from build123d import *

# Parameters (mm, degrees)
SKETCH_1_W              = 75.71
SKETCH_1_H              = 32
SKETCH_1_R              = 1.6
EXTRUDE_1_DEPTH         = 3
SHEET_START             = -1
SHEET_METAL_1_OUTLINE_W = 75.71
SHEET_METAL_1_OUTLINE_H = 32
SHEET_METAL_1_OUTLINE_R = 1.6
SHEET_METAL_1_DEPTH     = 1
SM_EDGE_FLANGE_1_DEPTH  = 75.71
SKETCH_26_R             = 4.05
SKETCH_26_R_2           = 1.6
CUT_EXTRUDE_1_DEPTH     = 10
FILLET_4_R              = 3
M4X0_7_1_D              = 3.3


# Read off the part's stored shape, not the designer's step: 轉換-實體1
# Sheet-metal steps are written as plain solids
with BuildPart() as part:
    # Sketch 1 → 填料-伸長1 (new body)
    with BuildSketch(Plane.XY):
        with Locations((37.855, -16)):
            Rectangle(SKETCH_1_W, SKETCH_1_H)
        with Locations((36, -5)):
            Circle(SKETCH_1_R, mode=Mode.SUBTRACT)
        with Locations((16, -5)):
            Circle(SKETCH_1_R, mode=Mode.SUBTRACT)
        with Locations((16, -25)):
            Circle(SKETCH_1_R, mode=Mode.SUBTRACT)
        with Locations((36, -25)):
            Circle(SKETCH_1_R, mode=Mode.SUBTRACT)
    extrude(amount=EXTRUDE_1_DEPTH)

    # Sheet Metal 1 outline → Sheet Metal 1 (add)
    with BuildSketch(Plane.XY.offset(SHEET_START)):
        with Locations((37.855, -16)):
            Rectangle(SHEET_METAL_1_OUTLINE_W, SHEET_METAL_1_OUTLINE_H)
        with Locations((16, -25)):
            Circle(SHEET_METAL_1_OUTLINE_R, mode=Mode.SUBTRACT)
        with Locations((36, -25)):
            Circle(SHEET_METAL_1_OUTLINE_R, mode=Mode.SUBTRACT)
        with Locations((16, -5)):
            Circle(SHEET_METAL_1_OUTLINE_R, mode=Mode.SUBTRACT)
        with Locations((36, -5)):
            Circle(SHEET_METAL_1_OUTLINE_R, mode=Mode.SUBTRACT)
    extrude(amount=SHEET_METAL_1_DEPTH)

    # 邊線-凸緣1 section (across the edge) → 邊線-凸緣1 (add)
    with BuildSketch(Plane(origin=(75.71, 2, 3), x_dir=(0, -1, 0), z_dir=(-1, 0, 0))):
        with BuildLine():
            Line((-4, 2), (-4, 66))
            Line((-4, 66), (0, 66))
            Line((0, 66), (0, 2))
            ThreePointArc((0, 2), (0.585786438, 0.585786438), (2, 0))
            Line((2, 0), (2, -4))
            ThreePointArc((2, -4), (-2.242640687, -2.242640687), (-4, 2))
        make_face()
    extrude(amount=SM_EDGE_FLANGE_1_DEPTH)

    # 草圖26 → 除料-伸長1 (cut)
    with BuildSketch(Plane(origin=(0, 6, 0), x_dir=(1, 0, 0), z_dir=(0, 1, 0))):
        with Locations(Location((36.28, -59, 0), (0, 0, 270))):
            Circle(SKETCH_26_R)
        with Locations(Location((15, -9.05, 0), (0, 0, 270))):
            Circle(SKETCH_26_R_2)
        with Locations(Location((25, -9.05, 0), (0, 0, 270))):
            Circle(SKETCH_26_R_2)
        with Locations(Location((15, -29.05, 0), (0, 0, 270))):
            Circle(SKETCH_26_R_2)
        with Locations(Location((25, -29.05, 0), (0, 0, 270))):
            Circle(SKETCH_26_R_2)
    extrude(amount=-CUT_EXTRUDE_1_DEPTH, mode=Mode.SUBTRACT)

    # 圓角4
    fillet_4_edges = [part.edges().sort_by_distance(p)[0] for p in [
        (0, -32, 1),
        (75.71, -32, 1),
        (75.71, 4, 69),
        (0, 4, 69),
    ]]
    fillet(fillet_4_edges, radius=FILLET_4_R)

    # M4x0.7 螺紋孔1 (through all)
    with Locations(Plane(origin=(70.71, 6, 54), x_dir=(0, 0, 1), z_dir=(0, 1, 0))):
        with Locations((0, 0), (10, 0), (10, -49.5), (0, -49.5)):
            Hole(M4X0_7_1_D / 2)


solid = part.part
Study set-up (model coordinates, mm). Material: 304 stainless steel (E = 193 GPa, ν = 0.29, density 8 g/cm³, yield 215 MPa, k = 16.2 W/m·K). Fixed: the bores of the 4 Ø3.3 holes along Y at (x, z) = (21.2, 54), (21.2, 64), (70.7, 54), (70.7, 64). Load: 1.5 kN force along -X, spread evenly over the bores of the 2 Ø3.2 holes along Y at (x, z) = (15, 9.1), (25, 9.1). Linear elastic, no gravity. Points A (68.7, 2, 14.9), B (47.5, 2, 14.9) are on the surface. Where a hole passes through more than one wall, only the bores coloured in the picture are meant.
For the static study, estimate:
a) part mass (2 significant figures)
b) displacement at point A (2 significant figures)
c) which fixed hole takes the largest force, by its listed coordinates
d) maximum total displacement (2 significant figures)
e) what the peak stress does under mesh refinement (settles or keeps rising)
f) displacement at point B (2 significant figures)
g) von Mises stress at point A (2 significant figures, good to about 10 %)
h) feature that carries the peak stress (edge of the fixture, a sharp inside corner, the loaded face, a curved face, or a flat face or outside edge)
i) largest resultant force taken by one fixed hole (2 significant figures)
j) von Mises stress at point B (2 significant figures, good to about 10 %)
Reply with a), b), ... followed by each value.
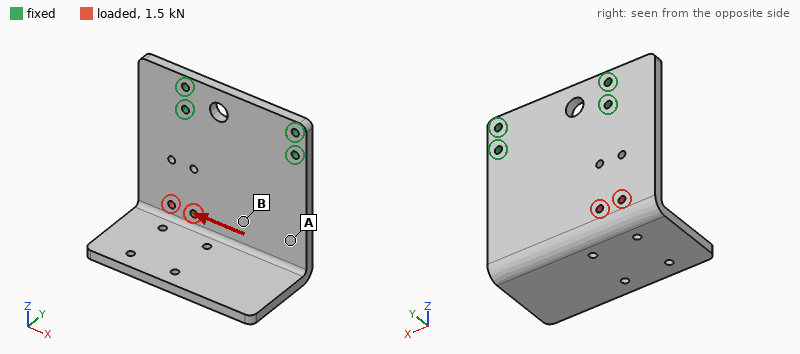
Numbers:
a) 240 g
b) 6.1 µm
c) (21.2, 54)
d) 10 µm
e) keeps rising
f) 5.9 µm
g) 4.6 MPa
h) edge of the fixture
i) 1.4 kN
j) 11 MPa
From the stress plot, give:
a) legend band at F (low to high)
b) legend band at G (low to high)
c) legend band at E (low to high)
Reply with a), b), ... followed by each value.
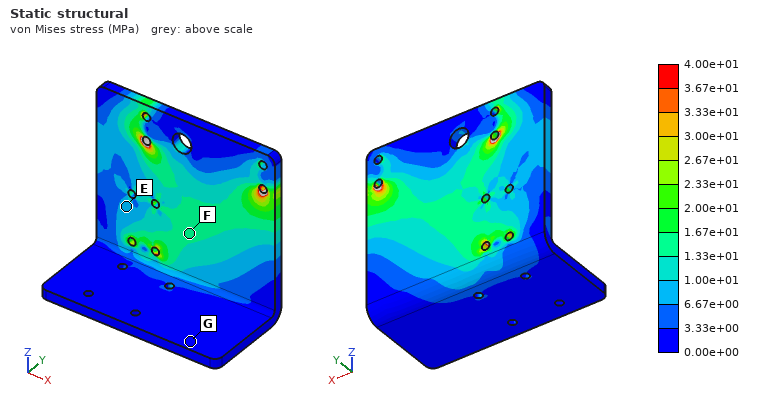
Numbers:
a) 1.33e+01 to 1.67e+01 MPa
b) 0.00e+00 to 3.33e+00 MPa
c) 6.67e+00 to 1.00e+01 MPa
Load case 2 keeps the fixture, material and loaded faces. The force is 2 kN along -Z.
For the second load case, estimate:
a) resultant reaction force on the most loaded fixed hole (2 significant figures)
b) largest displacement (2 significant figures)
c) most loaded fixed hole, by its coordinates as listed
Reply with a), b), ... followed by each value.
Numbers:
a) 1.4 kN
b) 6.2 µm
c) (21.2, 54)
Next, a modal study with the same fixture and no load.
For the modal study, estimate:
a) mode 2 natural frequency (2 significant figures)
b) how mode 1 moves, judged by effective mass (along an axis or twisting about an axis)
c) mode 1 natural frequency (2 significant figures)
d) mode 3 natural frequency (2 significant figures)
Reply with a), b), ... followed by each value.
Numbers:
a) 980 Hz
b) along Y
c) 490 Hz
d) 1700 Hz
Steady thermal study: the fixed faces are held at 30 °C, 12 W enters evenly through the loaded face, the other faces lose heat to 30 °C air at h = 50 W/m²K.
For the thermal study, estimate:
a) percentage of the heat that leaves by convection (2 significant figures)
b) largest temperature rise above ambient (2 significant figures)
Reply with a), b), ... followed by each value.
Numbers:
a) 89 %
b) 71 K
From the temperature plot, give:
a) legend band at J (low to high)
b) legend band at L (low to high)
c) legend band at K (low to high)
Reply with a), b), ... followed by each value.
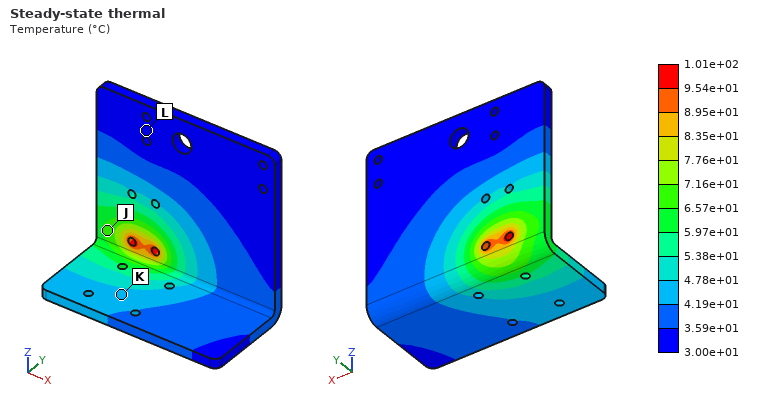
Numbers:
a) 6.57e+01 to 7.16e+01 °C
b) 3.00e+01 to 3.59e+01 °C
c) 4.19e+01 to 4.78e+01 °C
